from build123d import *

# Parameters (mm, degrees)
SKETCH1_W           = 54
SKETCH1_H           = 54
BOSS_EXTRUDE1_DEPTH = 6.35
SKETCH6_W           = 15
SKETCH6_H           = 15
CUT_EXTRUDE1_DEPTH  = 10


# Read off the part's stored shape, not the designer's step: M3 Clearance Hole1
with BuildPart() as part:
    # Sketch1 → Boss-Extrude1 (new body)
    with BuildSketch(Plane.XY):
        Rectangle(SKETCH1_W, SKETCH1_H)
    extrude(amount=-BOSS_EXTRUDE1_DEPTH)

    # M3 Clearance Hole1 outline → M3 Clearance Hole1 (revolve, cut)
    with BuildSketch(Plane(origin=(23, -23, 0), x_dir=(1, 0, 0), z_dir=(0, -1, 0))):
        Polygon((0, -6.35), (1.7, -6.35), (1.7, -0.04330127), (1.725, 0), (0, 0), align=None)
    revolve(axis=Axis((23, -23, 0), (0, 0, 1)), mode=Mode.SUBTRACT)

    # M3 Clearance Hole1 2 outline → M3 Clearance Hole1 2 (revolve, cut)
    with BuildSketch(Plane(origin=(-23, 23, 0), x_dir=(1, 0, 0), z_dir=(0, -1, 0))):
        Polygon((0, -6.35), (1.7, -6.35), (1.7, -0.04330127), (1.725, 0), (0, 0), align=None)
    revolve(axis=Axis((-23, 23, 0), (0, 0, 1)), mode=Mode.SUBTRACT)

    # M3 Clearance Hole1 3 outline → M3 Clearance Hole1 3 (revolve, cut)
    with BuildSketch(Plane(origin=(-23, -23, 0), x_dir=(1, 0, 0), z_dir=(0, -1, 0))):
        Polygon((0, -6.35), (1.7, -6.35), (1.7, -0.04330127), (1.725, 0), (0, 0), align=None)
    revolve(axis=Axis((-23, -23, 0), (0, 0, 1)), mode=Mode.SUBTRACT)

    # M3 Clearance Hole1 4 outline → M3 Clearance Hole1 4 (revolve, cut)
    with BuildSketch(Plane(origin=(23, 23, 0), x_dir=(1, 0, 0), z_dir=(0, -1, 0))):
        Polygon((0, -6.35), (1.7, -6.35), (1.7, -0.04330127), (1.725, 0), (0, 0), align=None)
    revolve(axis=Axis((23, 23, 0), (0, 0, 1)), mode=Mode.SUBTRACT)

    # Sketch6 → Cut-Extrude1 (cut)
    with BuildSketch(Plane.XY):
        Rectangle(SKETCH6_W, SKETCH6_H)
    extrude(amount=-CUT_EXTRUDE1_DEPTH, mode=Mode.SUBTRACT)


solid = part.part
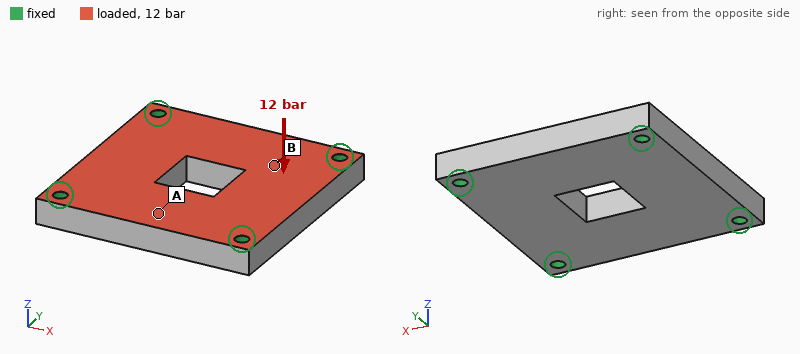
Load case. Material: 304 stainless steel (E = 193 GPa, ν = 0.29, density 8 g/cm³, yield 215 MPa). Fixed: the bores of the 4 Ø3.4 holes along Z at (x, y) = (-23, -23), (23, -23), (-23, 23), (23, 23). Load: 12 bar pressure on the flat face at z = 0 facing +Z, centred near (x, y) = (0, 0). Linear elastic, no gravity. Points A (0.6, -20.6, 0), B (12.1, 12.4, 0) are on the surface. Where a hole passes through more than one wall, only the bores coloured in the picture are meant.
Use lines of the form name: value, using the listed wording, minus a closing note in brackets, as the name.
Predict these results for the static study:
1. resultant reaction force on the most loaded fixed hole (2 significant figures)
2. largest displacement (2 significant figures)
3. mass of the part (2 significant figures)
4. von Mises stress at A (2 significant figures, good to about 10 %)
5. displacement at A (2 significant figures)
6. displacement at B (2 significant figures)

resultant reaction force on the most loaded fixed hole: 800 N
largest displacement: 12 µm
mass of the part: 130 g
von Mises stress at A: 21 MPa
displacement at A: 6.9 µm
displacement at B: 7.5 µm
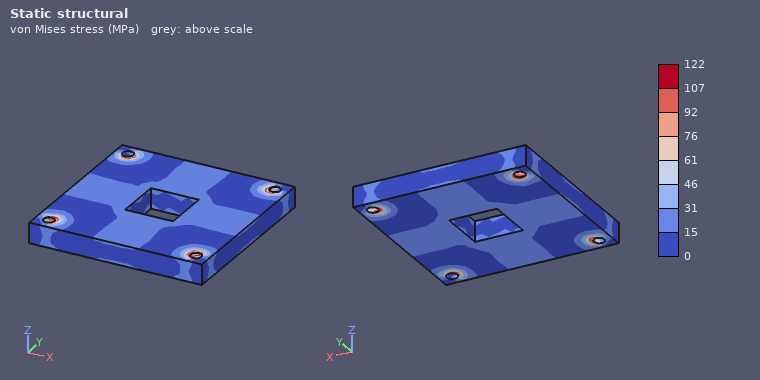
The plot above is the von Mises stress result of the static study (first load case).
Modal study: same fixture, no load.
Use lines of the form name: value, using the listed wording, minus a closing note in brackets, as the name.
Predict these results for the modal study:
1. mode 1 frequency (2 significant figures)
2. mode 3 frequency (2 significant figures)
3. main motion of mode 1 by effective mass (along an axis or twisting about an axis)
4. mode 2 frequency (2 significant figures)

mode 1 frequency: 8900 Hz
mode 3 frequency: 14 kHz
main motion of mode 1 by effective mass: along Z
mode 2 frequency: 14 kHz
